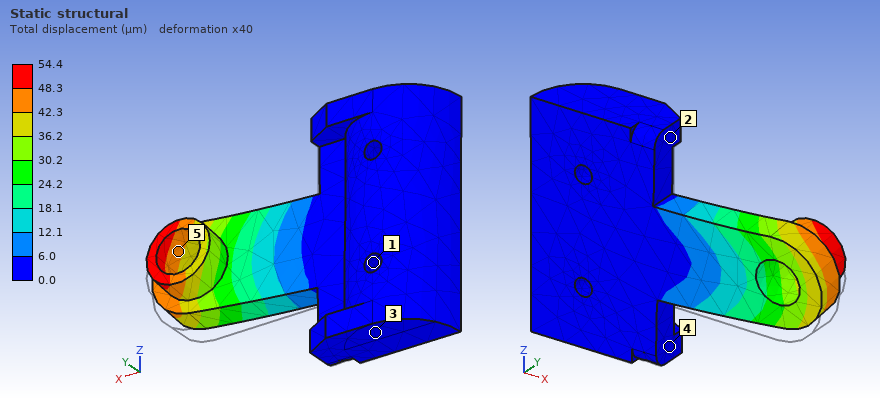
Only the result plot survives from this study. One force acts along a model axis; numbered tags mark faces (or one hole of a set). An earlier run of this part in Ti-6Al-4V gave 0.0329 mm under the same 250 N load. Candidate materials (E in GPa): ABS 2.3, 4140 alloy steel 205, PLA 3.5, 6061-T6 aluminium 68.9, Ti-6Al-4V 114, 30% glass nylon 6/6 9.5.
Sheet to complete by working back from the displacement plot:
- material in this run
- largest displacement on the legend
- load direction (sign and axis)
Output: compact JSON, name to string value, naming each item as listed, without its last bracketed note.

{"material in this run": "6061-T6 aluminium", "largest displacement on the legend": "54.4 µm", "load direction": "+Z"}
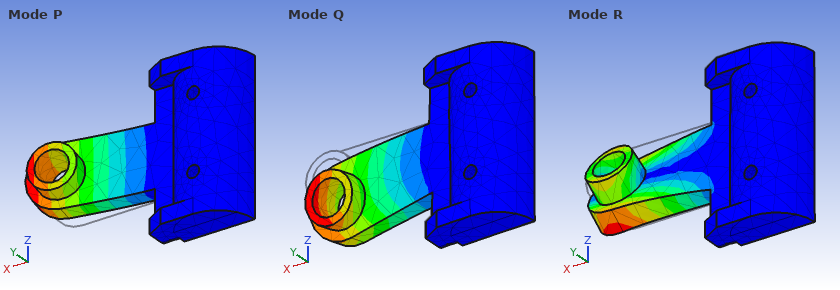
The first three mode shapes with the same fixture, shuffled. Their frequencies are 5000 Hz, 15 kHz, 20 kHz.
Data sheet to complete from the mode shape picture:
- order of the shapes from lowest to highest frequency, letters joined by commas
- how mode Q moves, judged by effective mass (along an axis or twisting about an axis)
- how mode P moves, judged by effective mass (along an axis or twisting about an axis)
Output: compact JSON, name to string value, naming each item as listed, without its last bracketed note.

{"order of the shapes from lowest to highest frequency, letters joined by commas": "P, Q, R", "how mode Q moves, judged by effective mass": "along Z", "how mode P moves, judged by effective mass": "along Y"}
